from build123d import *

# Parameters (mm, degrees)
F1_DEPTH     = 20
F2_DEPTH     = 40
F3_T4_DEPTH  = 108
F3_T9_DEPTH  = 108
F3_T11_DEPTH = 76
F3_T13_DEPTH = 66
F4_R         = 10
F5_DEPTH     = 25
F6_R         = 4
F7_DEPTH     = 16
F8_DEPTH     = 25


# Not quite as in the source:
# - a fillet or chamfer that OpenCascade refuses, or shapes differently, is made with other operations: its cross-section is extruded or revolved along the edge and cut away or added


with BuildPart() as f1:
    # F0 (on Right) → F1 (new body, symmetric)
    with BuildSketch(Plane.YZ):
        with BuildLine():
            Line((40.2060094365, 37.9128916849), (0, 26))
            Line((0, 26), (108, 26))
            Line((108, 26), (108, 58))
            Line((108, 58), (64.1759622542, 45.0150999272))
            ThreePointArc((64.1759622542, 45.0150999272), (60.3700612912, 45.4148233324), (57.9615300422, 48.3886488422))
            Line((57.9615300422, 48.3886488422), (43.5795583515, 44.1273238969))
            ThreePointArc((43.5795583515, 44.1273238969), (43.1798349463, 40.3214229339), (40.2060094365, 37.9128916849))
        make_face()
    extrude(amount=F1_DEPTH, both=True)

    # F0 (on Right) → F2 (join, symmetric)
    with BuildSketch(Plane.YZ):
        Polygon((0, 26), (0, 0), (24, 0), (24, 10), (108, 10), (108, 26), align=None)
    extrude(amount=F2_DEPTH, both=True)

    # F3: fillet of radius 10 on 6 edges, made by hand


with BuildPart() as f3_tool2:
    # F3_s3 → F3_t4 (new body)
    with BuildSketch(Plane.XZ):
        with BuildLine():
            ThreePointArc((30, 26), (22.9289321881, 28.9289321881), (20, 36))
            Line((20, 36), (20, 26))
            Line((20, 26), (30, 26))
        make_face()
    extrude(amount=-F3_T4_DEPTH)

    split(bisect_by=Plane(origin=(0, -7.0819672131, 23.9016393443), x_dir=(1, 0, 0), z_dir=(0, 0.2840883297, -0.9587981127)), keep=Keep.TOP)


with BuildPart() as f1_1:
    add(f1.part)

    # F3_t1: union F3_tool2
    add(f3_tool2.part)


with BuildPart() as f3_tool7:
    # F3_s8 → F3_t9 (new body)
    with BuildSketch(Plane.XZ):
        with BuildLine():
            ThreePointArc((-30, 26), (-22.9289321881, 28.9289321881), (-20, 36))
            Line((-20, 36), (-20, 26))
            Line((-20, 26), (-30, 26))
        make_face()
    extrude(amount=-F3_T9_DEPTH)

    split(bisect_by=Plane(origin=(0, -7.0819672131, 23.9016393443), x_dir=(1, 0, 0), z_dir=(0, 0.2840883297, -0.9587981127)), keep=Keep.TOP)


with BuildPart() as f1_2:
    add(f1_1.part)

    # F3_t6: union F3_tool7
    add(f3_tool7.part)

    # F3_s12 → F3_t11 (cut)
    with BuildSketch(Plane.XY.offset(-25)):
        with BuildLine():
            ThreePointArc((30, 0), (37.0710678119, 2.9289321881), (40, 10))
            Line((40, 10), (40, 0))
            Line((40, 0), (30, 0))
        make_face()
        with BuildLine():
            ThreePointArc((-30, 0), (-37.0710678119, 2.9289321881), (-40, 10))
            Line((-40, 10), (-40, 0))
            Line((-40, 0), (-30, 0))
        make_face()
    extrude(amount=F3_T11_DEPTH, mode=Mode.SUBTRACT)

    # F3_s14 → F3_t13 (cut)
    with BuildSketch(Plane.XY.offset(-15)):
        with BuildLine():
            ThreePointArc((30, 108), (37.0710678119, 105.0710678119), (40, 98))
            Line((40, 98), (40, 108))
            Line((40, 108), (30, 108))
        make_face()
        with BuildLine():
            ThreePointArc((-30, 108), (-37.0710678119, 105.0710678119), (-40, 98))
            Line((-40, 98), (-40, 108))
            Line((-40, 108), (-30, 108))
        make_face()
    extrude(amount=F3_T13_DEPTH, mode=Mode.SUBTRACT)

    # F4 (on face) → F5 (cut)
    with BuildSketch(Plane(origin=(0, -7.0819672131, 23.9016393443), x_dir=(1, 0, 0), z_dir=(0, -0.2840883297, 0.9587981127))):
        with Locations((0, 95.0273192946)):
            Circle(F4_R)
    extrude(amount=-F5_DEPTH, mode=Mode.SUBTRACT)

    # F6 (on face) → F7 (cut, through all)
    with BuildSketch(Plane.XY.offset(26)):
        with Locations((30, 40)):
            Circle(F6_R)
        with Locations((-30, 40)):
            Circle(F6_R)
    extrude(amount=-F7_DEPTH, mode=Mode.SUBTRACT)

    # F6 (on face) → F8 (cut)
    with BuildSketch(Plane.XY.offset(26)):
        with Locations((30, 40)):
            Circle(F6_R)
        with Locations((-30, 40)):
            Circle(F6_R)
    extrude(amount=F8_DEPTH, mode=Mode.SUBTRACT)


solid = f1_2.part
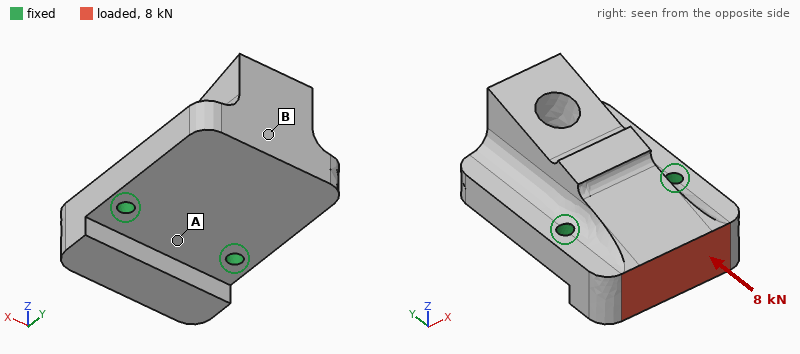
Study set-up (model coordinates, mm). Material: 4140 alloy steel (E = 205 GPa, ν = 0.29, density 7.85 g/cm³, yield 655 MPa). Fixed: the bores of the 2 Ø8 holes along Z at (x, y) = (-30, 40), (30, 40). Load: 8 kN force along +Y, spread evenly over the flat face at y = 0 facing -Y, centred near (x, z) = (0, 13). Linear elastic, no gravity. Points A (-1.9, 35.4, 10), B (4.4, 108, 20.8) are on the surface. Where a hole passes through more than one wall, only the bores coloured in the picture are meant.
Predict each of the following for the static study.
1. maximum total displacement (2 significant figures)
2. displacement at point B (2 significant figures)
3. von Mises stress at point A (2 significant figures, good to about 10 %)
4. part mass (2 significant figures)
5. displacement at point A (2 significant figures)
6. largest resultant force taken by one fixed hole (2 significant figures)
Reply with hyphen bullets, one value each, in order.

- 6.9 µm
- 3.1 µm
- 8.6 MPa
- 1.8 kg
- 1.6 µm
- 4.1 kN
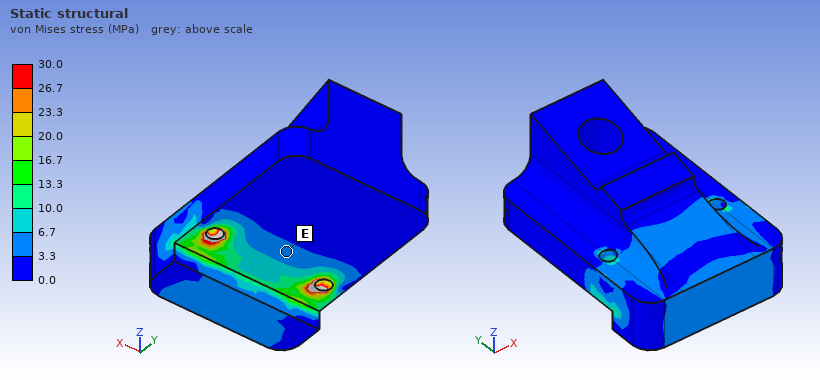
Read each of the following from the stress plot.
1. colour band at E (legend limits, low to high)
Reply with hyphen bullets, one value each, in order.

- 3.3 to 6.7 MPa
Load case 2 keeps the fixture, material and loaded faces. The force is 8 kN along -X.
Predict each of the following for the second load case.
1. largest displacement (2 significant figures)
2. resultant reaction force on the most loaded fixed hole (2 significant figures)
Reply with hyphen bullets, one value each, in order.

- 4.7 µm
- 6.4 kN
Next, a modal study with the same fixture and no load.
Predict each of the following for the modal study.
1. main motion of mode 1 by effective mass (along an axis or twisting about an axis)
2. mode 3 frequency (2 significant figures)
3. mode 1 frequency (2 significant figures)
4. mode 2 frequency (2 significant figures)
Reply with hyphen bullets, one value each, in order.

- along Z
- 6700 Hz
- 2300 Hz
- 6600 Hz
